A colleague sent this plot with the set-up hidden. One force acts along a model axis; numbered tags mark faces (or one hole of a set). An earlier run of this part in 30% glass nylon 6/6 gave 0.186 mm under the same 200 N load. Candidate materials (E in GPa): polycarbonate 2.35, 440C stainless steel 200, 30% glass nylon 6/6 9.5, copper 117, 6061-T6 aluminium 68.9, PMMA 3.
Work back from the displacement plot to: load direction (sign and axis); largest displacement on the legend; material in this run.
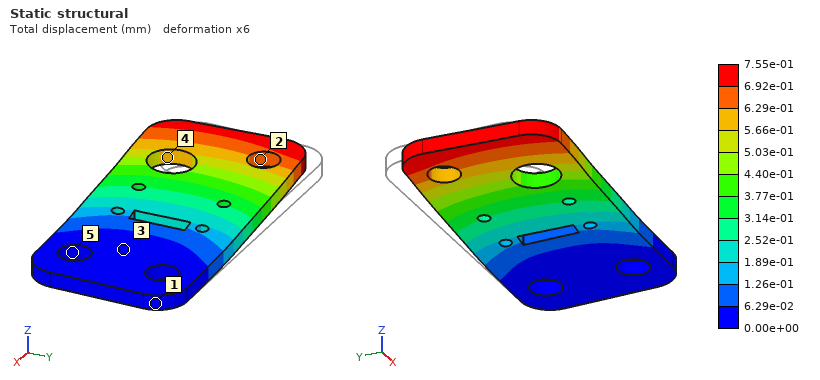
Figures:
-Y
7.55e-01 mm
polycarbonate
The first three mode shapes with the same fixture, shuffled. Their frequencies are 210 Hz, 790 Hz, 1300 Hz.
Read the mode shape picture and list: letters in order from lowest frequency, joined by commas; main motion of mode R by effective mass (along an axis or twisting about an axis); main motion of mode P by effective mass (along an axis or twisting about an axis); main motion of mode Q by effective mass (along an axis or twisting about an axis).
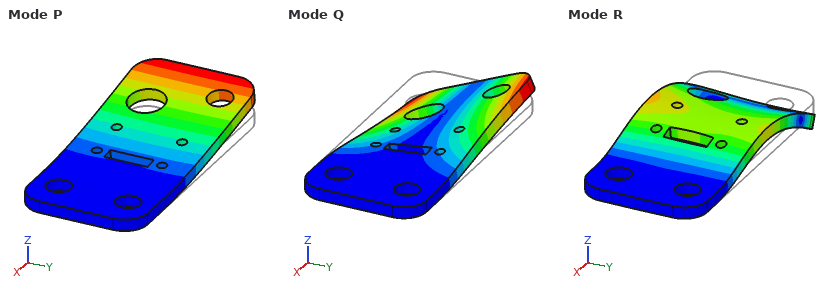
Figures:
P, Q, R
along Z
along Z
twisting about X
